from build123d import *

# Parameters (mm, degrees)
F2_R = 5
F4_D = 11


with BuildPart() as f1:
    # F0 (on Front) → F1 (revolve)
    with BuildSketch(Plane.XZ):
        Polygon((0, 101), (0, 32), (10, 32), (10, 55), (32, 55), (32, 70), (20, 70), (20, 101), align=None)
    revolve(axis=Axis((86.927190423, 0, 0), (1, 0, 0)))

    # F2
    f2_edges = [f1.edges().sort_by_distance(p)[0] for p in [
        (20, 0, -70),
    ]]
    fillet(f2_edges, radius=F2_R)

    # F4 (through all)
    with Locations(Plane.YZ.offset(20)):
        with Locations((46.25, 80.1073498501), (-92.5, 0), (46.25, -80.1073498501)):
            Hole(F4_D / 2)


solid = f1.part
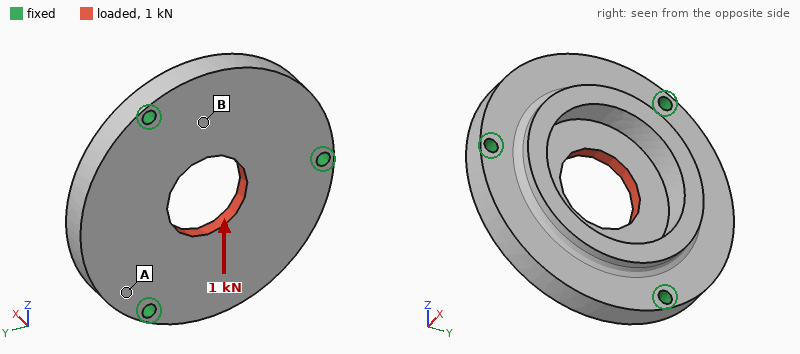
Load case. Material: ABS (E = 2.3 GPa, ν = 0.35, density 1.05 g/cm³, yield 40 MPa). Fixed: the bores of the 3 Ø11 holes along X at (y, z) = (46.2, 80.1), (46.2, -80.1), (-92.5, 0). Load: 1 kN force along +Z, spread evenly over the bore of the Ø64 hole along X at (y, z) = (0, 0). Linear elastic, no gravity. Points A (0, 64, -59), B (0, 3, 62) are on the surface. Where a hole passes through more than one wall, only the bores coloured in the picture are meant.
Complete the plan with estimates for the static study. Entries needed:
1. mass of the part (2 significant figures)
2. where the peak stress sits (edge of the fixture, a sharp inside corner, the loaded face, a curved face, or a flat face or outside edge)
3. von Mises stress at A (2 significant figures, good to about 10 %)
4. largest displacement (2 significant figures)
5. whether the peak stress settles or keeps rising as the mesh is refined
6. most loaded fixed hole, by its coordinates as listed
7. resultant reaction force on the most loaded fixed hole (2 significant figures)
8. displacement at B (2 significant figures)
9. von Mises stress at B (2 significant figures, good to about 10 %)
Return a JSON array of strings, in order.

["610 g", "edge of the fixture", "0.19 MPa", "27 µm", "keeps rising", "(-92.5, 0)", "360 N", "17 µm", "0.46 MPa"]
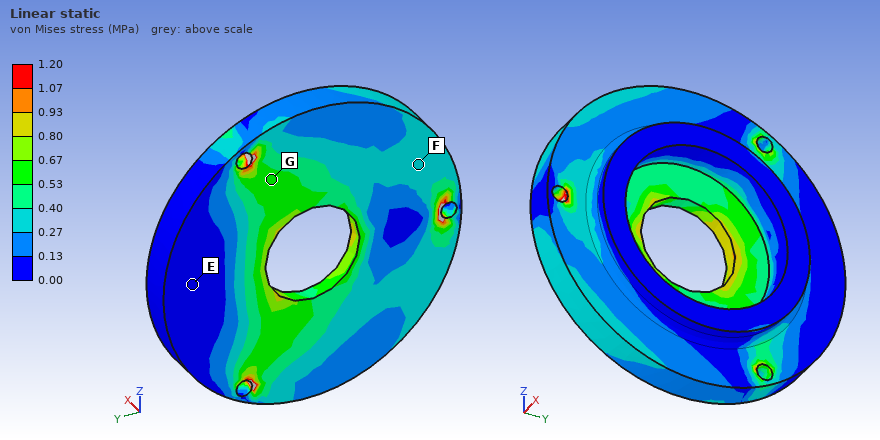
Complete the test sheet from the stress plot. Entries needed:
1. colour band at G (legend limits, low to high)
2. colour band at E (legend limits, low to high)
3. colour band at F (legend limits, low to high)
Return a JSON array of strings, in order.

["0.53 to 0.67 MPa", "0.00 to 0.13 MPa", "0.27 to 0.40 MPa"]
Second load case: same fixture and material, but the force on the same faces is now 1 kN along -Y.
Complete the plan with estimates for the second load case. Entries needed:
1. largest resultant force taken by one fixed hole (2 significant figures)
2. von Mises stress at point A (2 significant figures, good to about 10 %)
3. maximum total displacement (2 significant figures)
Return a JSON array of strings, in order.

["350 N", "0.38 MPa", "30 µm"]
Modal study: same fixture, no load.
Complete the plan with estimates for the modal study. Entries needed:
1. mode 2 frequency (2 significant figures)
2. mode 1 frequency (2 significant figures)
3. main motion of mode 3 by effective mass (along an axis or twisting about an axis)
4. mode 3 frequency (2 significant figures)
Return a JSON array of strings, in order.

["810 Hz", "810 Hz", "along X", "960 Hz"]
